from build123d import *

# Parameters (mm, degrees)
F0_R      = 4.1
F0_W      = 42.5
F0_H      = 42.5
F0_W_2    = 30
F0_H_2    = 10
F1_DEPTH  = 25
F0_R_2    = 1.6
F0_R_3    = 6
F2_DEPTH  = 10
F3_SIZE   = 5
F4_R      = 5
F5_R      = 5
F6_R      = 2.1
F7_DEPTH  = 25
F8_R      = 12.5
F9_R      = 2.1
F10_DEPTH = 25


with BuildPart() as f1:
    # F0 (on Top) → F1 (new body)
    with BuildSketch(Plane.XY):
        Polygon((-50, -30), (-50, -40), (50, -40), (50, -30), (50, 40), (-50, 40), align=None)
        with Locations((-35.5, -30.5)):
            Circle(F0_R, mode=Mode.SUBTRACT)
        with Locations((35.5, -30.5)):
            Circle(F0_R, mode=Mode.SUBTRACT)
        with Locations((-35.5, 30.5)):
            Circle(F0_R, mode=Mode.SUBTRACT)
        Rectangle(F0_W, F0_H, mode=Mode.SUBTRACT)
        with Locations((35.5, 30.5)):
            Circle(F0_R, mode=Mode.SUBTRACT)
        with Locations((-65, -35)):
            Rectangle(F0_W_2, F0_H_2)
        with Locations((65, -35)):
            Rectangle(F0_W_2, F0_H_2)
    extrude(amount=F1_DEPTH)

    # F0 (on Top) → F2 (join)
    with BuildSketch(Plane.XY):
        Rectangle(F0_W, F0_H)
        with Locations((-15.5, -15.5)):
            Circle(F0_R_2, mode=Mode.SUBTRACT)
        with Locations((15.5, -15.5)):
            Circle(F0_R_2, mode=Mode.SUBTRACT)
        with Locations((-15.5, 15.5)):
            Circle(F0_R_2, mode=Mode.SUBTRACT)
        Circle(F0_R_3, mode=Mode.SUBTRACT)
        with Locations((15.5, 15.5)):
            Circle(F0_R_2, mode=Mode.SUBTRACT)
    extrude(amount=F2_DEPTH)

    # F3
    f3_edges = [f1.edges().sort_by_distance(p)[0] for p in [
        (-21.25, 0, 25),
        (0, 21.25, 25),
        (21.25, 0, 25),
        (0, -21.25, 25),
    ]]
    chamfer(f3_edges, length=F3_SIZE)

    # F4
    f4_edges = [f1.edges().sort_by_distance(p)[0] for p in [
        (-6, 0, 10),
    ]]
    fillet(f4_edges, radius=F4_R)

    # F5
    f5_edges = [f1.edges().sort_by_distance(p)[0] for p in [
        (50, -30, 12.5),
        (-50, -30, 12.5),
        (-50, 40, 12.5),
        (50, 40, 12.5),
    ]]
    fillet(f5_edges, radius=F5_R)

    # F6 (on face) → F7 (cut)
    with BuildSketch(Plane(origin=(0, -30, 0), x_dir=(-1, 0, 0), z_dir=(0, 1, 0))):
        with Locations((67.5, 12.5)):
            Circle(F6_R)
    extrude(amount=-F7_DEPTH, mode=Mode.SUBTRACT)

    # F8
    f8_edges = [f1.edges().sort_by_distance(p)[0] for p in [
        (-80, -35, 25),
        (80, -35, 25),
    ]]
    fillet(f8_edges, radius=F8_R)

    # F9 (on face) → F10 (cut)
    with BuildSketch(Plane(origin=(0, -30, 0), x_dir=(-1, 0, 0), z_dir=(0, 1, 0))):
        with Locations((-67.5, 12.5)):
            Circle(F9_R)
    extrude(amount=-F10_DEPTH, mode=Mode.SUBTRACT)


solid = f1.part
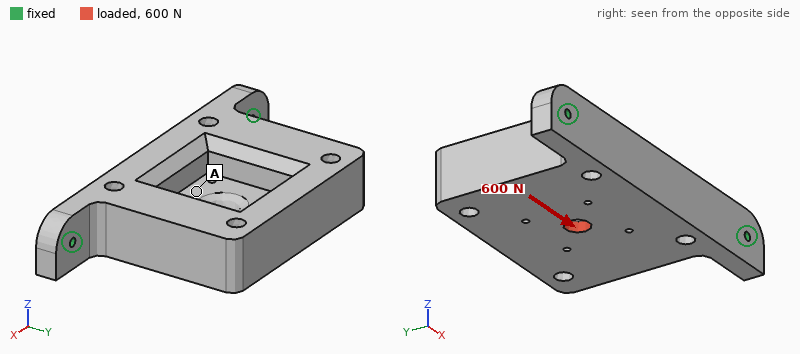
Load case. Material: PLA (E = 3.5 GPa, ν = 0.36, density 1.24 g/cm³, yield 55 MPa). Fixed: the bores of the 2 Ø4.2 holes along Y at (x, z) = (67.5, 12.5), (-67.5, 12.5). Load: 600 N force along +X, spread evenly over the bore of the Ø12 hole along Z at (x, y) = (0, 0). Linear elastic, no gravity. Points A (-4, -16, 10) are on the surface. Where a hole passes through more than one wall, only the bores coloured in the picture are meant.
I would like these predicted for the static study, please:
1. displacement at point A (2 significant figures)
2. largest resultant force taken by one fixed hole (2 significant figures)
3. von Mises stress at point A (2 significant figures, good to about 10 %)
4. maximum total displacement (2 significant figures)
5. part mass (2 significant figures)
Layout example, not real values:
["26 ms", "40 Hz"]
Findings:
["27 µm", "350 N", "1.0 MPa", "74 µm", "220 g"]
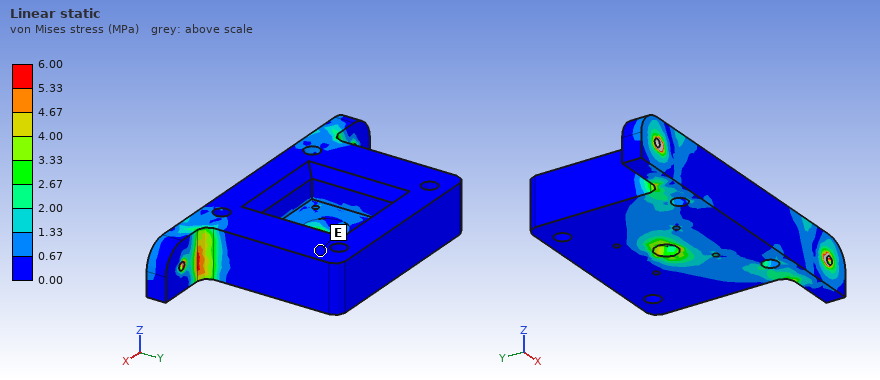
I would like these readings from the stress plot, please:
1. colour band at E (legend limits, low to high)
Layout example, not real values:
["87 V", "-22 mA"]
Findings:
["0.00 to 0.67 MPa"]
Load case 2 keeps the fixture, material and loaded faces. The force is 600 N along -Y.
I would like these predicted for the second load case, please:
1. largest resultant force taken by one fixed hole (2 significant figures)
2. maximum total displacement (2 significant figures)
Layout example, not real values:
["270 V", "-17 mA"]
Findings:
["350 N", "0.60 mm"]
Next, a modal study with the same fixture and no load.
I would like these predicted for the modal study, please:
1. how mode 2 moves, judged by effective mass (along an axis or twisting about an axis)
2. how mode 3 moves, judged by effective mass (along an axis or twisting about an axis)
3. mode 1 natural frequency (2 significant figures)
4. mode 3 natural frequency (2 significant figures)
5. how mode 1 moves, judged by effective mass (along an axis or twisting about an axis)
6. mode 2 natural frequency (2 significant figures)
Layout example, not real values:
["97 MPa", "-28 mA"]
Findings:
["along Y", "along X", "230 Hz", "1100 Hz", "along Z", "1000 Hz"]
